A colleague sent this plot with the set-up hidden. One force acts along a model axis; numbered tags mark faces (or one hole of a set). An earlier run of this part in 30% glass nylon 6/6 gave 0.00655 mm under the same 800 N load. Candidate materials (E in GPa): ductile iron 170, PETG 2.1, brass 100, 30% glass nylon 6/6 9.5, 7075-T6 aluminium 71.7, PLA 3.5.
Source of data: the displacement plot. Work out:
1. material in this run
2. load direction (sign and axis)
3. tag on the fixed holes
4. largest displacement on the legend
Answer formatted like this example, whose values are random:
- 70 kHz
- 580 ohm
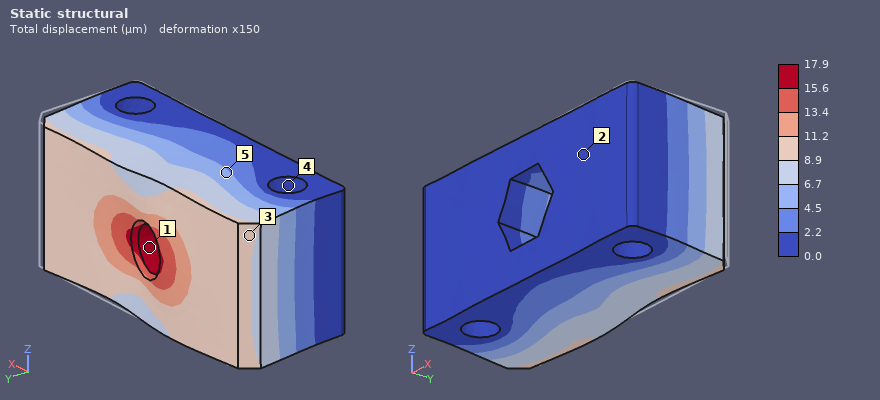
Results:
- PLA
- -X
- 4
- 17.9 µm
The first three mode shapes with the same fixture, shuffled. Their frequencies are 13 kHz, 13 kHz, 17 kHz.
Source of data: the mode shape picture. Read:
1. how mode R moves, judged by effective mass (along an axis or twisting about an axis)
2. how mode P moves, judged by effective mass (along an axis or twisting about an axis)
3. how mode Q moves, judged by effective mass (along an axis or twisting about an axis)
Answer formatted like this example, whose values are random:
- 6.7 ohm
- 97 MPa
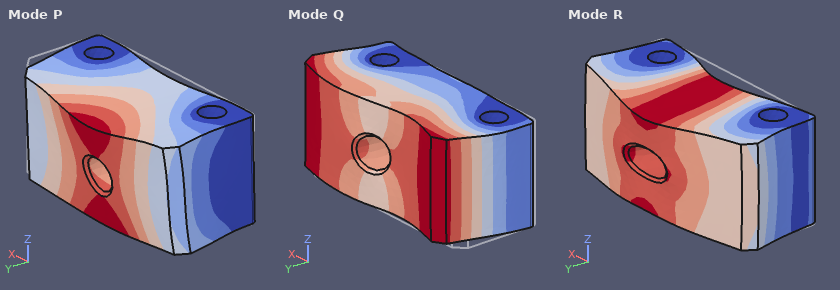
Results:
- along Y
- along Z
- along X
